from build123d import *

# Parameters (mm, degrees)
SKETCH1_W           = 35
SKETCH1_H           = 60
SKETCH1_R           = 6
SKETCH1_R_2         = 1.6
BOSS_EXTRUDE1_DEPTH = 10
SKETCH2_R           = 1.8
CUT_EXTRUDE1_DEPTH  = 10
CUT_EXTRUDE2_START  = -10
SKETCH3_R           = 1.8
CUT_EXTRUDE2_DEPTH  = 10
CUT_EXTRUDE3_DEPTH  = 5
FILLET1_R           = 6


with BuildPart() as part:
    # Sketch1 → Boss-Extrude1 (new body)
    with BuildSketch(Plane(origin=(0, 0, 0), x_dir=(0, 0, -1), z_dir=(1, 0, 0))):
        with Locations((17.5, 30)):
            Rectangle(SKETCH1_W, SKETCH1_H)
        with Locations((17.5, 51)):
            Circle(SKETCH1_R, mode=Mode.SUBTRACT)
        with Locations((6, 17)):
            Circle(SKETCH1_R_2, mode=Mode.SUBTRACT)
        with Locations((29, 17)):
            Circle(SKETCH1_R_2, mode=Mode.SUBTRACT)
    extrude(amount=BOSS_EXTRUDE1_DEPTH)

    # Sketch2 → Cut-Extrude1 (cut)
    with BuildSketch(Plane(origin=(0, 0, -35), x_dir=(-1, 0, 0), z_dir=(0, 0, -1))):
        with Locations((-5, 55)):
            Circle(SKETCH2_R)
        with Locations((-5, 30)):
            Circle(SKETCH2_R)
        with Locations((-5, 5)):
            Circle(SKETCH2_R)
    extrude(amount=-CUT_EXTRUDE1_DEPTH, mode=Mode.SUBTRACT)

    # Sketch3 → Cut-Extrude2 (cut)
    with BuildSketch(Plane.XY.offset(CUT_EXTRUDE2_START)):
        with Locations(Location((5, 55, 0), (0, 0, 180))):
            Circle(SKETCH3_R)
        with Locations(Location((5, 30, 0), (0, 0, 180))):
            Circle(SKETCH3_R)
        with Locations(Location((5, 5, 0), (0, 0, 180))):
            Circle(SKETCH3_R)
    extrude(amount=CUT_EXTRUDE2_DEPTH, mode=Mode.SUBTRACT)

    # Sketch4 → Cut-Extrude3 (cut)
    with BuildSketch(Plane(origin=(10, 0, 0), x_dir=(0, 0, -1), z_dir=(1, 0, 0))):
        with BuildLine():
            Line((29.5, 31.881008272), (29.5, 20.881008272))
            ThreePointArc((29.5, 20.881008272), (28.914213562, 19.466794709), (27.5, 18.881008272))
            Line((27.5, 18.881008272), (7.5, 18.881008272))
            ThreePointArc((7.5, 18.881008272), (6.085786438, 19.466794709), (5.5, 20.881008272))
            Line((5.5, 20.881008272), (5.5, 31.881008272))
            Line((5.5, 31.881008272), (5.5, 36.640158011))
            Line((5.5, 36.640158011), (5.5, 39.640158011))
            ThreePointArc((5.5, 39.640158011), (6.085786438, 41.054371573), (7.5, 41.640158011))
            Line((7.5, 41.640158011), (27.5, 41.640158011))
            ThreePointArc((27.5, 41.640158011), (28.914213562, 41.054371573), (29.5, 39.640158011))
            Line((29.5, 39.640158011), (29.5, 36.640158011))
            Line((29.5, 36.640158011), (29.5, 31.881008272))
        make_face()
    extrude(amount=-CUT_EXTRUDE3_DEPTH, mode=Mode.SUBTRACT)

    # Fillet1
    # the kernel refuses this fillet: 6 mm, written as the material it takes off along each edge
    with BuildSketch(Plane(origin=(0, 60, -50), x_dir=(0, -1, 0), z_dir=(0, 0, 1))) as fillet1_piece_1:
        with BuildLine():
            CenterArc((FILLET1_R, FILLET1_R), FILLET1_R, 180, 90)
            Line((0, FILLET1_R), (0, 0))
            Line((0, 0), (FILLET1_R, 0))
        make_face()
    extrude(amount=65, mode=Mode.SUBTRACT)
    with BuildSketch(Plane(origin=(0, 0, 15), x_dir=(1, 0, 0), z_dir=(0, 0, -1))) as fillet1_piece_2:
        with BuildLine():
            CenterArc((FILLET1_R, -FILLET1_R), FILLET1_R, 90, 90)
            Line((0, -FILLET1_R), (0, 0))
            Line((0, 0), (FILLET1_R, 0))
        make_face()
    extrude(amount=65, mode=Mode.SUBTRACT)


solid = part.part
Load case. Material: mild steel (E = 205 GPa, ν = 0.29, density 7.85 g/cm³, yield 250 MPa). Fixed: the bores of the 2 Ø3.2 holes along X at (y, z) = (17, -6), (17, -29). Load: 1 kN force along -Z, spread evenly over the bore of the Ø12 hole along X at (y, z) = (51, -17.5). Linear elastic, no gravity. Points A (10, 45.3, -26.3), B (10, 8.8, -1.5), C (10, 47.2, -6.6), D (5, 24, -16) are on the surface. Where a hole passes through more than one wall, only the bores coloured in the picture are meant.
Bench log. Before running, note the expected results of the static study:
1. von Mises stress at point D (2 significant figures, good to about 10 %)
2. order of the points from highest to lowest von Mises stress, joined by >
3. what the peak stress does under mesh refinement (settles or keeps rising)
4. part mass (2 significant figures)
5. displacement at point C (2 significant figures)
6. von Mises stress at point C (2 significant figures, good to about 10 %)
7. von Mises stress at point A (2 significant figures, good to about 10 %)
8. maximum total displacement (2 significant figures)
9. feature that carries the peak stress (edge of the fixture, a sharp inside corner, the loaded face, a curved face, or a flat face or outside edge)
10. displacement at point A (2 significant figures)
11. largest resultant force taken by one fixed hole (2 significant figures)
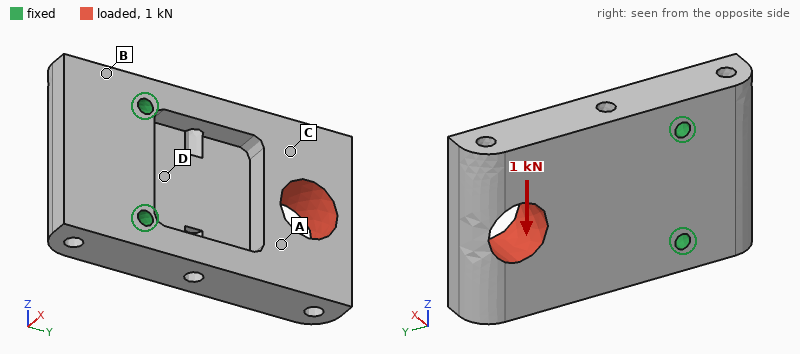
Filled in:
18 MPa
D > C > A > B
keeps rising
120 g
7.2 µm
11 MPa
8.4 MPa
11 µm
edge of the fixture
6.6 µm
1.4 kN
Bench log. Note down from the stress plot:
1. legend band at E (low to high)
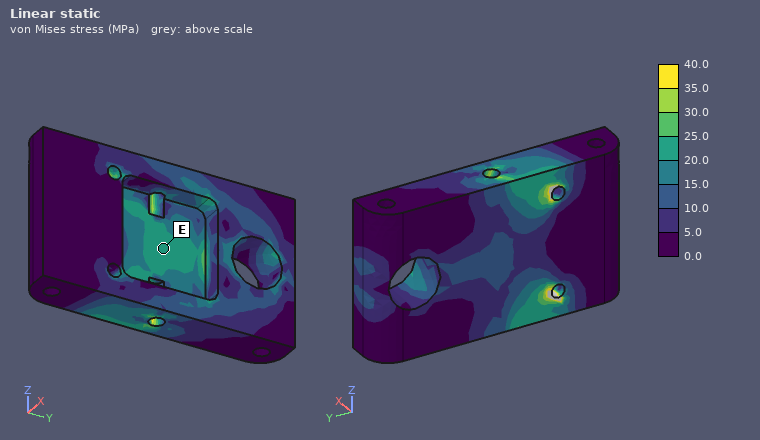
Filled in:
20.0 to 25.0 MPa
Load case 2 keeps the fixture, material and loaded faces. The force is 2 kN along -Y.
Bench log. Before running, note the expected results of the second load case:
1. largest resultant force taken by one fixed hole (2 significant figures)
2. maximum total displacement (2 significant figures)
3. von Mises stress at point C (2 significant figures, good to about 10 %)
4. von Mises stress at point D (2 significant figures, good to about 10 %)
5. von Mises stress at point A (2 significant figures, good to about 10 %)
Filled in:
1.0 kN
10 µm
13 MPa
12 MPa
14 MPa
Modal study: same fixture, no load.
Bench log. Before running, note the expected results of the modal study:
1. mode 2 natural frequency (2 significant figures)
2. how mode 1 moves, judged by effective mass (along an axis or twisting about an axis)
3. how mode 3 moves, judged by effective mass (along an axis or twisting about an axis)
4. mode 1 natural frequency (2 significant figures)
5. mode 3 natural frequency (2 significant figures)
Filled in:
7000 Hz
along X
along Z
3400 Hz
10 kHz
